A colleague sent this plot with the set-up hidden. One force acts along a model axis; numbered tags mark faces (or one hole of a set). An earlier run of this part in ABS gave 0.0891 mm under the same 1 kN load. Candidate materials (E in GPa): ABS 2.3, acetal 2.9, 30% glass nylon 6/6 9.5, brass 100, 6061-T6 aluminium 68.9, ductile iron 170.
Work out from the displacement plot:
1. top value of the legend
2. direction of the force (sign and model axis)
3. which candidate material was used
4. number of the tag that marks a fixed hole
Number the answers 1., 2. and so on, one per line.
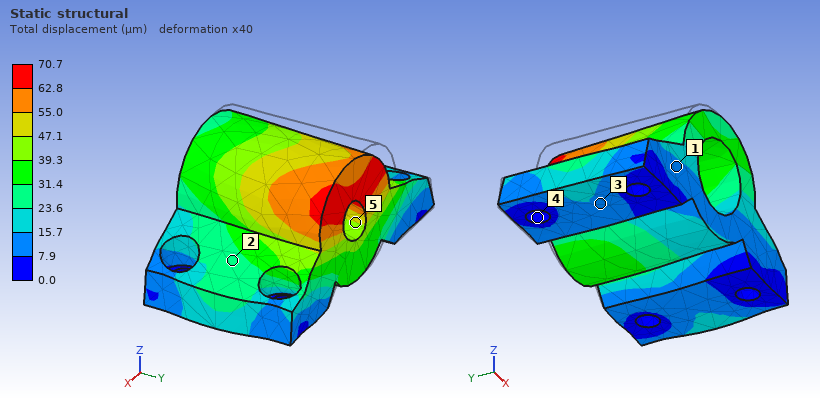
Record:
1. 70.7 µm
2. +X
3. acetal
4. 4
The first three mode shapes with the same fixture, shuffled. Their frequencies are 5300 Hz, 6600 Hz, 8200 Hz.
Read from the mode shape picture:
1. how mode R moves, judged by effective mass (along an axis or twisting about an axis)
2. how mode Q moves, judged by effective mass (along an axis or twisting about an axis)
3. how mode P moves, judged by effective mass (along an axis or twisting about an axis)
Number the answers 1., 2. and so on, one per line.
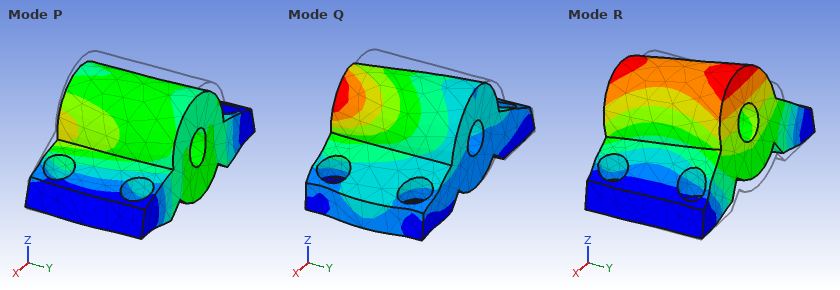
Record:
1. along Y
2. along X
3. along Z
